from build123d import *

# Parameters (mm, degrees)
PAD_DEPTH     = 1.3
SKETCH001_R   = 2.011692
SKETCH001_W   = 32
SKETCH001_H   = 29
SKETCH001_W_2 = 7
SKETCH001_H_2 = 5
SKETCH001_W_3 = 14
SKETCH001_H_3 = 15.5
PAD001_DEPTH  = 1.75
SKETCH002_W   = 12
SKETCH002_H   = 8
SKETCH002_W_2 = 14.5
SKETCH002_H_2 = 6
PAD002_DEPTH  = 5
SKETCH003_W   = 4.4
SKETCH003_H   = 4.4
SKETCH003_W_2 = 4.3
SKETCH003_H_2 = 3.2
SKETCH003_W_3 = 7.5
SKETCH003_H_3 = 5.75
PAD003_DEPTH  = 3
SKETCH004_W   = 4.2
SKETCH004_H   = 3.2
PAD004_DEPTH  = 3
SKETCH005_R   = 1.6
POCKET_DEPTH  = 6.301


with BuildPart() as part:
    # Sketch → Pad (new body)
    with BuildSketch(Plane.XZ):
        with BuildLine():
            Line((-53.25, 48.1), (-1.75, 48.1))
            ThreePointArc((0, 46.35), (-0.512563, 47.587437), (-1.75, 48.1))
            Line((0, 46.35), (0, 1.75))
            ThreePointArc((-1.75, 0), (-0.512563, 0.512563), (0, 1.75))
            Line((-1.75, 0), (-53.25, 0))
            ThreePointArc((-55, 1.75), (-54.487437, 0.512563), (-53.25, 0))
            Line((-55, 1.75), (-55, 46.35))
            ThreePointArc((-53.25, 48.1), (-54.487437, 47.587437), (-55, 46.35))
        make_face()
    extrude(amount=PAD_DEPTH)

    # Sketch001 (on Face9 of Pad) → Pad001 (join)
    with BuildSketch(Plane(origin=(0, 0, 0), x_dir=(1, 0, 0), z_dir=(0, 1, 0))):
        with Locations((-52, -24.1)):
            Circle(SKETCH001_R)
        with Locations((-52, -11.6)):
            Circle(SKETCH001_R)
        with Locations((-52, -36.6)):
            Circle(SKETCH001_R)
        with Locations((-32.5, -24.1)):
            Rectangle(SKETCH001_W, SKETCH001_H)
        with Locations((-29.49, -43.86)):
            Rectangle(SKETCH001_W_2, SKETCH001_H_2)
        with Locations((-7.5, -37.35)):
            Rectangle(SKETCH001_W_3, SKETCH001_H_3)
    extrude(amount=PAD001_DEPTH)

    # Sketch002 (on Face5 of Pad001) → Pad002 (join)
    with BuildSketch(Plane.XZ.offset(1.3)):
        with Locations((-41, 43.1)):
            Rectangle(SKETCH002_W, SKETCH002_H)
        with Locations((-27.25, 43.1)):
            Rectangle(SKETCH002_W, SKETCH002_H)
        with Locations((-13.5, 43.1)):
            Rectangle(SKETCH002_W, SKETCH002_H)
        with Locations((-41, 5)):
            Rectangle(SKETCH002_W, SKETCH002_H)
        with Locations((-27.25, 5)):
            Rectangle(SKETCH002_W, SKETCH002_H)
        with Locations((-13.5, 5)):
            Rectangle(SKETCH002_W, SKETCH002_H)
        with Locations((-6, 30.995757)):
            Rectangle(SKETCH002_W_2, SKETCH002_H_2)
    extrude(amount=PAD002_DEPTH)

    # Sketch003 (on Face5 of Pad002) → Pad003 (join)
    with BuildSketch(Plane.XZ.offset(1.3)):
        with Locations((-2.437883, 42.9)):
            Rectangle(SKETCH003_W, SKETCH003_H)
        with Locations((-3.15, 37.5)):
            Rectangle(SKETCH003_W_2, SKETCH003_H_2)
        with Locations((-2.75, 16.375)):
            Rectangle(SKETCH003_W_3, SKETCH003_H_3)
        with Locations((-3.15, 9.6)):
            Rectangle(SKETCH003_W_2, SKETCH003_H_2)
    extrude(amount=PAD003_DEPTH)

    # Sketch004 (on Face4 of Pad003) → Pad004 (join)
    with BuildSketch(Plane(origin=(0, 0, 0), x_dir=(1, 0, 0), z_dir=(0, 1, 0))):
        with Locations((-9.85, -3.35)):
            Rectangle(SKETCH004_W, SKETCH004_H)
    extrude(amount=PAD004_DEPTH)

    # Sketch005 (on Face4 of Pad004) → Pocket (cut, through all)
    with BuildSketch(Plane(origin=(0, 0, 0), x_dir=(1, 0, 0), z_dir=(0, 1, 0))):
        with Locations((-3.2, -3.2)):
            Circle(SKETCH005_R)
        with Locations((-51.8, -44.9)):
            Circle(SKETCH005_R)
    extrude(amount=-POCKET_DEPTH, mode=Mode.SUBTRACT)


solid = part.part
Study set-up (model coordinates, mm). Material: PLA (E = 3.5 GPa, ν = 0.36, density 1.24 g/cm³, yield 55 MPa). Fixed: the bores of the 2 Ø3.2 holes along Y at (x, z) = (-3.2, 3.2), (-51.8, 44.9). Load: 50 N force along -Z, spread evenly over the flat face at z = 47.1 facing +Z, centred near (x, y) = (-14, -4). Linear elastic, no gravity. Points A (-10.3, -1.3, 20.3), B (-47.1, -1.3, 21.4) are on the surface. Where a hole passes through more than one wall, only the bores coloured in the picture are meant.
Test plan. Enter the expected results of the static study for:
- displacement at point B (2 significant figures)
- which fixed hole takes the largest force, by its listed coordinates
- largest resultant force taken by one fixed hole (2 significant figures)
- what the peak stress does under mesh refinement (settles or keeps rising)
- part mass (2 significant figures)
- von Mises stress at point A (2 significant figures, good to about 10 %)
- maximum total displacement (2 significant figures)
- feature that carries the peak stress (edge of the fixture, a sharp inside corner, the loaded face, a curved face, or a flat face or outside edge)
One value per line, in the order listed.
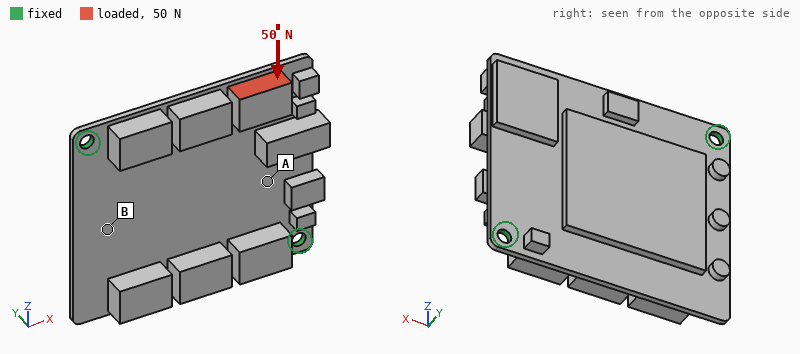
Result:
0.25 mm
(-3.2, 3.2)
35 N
keeps rising
11 g
2.5 MPa
0.78 mm
edge of the fixture
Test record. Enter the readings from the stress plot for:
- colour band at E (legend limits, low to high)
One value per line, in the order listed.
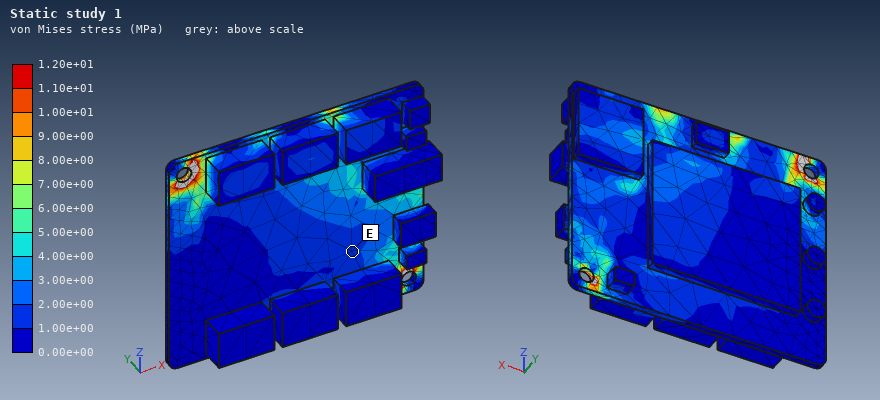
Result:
1.00e+00 to 2.00e+00 MPa
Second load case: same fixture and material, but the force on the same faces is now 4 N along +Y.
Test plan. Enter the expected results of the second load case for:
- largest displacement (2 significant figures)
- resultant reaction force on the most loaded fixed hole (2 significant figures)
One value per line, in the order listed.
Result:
0.73 mm
4.3 N
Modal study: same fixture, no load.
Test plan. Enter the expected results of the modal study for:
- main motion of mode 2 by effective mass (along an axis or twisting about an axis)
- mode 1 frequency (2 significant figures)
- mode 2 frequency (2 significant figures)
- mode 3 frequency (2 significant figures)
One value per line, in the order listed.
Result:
along Y
240 Hz
440 Hz
1200 Hz
